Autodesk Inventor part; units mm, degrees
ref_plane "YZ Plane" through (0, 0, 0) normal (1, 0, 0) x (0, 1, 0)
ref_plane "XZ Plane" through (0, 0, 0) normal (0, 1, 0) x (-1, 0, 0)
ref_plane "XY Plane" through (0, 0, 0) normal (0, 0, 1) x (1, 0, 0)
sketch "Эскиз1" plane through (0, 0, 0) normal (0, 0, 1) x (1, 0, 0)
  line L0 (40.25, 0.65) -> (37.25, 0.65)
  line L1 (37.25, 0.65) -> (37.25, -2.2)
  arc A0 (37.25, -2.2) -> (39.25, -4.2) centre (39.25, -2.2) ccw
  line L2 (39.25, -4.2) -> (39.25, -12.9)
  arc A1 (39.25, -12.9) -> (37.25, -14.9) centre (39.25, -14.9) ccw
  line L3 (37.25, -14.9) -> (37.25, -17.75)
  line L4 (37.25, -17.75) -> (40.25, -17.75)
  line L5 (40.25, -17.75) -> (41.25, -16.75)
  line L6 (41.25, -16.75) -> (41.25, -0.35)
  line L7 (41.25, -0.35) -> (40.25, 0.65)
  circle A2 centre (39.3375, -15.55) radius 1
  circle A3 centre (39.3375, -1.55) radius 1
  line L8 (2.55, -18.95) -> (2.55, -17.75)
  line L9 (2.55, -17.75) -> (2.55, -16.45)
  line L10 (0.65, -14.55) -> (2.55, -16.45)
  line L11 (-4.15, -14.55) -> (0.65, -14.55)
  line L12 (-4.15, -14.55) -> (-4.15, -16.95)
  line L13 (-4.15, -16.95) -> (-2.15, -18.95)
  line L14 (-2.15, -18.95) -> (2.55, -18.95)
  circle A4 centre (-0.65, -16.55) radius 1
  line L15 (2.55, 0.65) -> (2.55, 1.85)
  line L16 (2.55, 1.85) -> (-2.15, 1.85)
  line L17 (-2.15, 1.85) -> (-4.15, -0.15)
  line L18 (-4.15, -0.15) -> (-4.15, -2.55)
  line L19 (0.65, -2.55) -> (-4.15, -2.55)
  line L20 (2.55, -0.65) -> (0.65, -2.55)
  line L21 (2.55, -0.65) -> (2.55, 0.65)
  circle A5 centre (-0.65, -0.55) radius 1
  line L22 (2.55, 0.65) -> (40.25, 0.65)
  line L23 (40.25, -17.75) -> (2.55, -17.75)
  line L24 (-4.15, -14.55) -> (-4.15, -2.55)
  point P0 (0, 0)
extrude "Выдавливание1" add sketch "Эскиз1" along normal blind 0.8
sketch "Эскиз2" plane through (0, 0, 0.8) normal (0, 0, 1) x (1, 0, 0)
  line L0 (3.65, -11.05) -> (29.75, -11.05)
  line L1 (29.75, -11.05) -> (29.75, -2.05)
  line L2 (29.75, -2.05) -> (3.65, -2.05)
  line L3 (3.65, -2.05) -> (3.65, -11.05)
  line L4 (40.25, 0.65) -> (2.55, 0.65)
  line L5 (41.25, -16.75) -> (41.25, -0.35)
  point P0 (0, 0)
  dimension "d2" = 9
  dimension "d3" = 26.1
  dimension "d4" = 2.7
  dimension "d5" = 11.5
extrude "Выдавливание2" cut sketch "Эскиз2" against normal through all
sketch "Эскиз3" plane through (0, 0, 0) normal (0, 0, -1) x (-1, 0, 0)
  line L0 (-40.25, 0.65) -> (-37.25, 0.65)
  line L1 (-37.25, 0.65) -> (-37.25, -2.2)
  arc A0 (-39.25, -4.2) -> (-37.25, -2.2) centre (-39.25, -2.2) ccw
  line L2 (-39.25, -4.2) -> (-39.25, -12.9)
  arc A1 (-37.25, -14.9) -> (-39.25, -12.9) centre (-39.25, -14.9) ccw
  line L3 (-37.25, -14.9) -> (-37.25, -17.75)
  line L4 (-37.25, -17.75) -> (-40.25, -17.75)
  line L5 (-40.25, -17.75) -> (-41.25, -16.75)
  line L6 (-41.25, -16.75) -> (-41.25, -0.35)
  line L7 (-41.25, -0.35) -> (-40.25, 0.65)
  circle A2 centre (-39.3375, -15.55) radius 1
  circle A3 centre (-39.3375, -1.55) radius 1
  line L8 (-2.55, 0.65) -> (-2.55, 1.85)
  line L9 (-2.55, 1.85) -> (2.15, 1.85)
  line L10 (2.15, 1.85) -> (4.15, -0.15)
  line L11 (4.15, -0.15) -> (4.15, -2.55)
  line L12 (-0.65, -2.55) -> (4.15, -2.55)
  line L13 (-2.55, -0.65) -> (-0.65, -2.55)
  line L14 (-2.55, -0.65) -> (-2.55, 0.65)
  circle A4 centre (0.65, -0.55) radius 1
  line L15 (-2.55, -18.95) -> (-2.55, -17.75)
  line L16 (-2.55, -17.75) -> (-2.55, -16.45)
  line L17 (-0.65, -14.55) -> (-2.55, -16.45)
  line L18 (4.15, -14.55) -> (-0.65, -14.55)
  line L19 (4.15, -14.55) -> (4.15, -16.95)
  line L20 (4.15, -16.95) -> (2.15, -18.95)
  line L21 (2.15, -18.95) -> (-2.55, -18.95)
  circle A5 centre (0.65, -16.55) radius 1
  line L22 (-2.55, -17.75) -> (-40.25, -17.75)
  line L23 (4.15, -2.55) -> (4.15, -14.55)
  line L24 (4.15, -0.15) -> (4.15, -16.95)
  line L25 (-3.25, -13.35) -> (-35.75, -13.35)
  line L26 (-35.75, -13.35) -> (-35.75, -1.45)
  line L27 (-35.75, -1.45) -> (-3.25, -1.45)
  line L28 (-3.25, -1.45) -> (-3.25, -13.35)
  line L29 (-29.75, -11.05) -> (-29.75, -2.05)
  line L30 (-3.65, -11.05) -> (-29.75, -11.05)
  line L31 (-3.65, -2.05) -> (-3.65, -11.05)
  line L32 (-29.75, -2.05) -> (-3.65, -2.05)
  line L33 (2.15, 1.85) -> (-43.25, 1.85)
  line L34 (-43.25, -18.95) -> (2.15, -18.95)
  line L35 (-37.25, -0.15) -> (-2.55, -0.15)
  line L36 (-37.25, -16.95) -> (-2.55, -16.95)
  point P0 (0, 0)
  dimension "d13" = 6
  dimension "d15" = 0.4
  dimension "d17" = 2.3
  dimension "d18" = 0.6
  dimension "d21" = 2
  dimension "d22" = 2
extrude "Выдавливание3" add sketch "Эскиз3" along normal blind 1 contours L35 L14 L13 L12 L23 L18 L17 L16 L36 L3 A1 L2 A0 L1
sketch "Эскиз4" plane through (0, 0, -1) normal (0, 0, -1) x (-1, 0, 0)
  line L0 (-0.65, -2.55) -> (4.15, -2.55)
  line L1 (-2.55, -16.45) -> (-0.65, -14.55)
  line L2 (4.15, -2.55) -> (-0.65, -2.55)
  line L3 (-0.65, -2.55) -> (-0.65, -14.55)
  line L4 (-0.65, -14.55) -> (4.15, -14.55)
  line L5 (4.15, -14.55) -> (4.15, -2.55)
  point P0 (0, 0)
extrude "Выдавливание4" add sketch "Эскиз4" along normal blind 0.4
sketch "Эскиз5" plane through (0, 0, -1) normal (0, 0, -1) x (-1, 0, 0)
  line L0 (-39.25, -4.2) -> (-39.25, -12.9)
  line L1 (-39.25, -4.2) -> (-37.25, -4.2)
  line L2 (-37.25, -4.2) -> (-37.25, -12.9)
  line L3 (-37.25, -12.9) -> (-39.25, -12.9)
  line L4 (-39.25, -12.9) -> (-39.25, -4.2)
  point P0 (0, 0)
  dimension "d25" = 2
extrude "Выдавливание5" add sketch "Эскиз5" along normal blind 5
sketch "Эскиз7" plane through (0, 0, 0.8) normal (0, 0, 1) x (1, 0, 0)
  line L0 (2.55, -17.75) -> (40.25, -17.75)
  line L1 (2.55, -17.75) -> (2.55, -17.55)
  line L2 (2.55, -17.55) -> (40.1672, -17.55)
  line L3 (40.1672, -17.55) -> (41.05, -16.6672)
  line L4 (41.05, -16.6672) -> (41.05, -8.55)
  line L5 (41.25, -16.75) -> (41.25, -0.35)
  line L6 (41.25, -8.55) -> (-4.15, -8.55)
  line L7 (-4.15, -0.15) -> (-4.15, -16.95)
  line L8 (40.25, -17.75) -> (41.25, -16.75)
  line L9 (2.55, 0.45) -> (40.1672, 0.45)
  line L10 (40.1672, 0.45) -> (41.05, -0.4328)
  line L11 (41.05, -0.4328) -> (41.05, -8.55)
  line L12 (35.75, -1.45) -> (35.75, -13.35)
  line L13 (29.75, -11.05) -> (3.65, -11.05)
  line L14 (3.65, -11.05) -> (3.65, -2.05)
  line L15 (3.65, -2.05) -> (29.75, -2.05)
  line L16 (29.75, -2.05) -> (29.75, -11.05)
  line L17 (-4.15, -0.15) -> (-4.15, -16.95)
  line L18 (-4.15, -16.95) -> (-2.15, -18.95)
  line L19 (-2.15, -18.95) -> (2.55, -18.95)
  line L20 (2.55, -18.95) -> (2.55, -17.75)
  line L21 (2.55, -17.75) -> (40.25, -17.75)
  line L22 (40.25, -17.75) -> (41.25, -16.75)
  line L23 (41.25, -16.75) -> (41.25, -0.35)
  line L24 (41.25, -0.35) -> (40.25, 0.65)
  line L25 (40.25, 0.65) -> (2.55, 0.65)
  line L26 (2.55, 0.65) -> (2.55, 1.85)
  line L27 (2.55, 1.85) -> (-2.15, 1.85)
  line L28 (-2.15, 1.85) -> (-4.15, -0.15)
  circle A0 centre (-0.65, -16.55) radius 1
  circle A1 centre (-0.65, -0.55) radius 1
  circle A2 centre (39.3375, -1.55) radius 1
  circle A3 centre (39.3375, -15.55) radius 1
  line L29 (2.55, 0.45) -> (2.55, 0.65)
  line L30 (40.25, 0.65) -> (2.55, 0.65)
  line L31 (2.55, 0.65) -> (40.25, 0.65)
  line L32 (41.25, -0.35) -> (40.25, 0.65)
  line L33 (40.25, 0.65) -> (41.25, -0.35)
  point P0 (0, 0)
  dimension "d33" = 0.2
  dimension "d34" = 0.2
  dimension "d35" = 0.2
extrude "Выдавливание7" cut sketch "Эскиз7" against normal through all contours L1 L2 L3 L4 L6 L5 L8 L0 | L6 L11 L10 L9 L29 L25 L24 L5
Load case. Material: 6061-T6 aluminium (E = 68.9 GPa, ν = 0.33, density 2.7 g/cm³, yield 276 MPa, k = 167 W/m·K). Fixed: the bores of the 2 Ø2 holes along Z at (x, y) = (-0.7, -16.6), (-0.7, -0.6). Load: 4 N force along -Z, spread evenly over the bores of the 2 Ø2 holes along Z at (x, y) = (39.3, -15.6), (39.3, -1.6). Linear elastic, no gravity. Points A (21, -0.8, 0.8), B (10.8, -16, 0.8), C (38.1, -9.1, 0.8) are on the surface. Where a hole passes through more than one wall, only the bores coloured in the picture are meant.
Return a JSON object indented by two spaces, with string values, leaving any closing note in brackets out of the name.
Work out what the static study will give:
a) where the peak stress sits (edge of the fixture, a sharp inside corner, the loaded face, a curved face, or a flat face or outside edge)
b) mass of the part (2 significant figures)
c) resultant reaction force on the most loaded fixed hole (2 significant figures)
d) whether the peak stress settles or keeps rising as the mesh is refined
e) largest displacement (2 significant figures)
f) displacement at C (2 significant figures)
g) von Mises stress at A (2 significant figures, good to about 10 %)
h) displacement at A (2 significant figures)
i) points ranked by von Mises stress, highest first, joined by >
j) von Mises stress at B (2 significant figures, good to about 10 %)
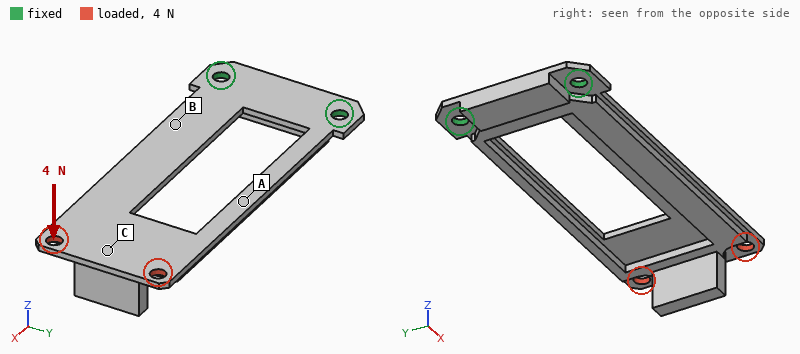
{
  "where the peak stress sits": "edge of the fixture",
  "mass of the part": "2.4 g",
  "resultant reaction force on the most loaded fixed hole": "11 N",
  "whether the peak stress settles or keeps rising as the mesh is refined": "keeps rising",
  "largest displacement": "0.51 mm",
  "displacement at C": "0.45 mm",
  "von Mises stress at A": "17 MPa",
  "displacement at A": "0.19 mm",
  "points ranked by von Mises stress, highest first, joined by >": "B > A > C",
  "von Mises stress at B": "29 MPa"
}
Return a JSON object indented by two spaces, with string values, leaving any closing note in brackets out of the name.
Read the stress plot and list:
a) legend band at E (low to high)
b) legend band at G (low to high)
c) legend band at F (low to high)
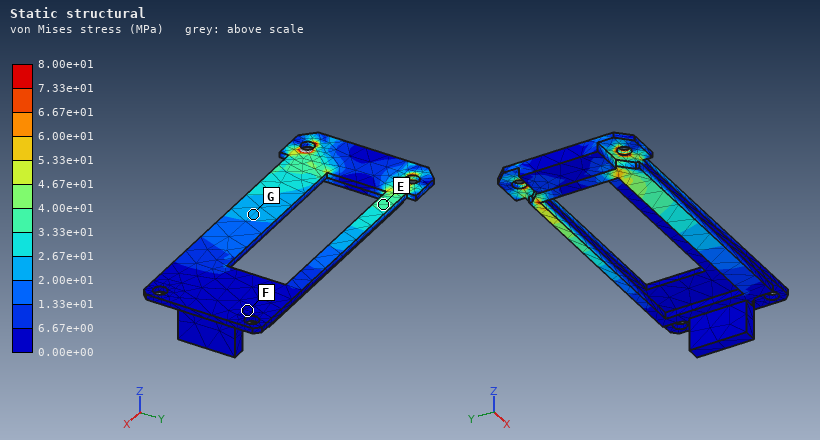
{
  "legend band at E": "3.33e+01 to 4.00e+01 MPa",
  "legend band at G": "2.00e+01 to 2.67e+01 MPa",
  "legend band at F": "0.00e+00 to 6.67e+00 MPa"
}
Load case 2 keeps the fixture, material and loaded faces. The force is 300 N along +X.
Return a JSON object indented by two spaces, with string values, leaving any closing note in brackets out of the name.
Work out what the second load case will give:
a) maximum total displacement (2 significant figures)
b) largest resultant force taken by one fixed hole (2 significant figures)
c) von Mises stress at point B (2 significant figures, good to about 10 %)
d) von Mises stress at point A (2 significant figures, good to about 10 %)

{
  "maximum total displacement": "0.37 mm",
  "largest resultant force taken by one fixed hole": "150 N",
  "von Mises stress at point B": "43 MPa",
  "von Mises stress at point A": "67 MPa"
}
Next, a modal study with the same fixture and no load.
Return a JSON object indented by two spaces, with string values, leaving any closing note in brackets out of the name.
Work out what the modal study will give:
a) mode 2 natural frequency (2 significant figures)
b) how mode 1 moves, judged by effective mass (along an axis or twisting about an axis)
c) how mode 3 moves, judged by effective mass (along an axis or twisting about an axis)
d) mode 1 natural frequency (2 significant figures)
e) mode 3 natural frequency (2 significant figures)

{
  "mode 2 natural frequency": "2300 Hz",
  "how mode 1 moves, judged by effective mass": "along Z",
  "how mode 3 moves, judged by effective mass": "along Y",
  "mode 1 natural frequency": "520 Hz",
  "mode 3 natural frequency": "3200 Hz"
}
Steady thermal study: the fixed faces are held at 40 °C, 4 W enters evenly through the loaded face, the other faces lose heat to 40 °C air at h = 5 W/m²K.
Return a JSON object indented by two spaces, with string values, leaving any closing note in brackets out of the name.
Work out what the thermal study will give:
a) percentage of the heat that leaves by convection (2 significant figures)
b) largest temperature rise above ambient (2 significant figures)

{
  "percentage of the heat that leaves by convection": "7.6 %",
  "largest temperature rise above ambient": "78 K"
}
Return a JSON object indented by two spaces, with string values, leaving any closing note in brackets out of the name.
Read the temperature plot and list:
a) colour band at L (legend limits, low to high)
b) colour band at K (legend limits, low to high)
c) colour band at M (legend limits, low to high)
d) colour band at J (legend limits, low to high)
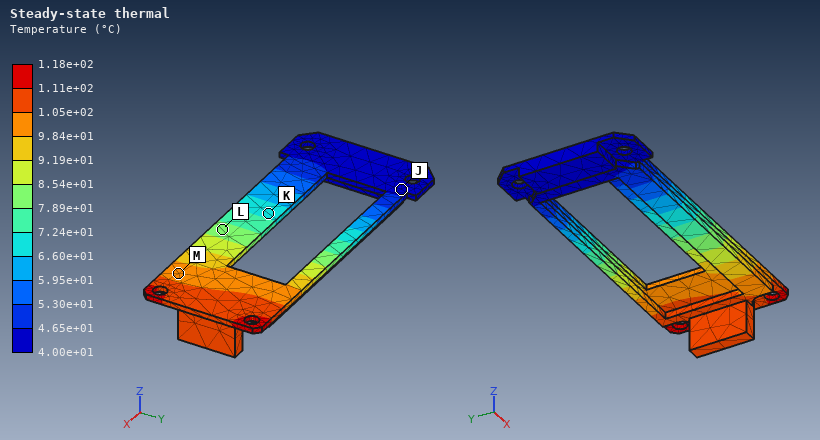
{
  "colour band at L": "7.89e+01 to 8.54e+01 °C",
  "colour band at K": "6.60e+01 to 7.24e+01 °C",
  "colour band at M": "9.84e+01 to 1.05e+02 °C",
  "colour band at J": "4.00e+01 to 4.65e+01 °C"
}
